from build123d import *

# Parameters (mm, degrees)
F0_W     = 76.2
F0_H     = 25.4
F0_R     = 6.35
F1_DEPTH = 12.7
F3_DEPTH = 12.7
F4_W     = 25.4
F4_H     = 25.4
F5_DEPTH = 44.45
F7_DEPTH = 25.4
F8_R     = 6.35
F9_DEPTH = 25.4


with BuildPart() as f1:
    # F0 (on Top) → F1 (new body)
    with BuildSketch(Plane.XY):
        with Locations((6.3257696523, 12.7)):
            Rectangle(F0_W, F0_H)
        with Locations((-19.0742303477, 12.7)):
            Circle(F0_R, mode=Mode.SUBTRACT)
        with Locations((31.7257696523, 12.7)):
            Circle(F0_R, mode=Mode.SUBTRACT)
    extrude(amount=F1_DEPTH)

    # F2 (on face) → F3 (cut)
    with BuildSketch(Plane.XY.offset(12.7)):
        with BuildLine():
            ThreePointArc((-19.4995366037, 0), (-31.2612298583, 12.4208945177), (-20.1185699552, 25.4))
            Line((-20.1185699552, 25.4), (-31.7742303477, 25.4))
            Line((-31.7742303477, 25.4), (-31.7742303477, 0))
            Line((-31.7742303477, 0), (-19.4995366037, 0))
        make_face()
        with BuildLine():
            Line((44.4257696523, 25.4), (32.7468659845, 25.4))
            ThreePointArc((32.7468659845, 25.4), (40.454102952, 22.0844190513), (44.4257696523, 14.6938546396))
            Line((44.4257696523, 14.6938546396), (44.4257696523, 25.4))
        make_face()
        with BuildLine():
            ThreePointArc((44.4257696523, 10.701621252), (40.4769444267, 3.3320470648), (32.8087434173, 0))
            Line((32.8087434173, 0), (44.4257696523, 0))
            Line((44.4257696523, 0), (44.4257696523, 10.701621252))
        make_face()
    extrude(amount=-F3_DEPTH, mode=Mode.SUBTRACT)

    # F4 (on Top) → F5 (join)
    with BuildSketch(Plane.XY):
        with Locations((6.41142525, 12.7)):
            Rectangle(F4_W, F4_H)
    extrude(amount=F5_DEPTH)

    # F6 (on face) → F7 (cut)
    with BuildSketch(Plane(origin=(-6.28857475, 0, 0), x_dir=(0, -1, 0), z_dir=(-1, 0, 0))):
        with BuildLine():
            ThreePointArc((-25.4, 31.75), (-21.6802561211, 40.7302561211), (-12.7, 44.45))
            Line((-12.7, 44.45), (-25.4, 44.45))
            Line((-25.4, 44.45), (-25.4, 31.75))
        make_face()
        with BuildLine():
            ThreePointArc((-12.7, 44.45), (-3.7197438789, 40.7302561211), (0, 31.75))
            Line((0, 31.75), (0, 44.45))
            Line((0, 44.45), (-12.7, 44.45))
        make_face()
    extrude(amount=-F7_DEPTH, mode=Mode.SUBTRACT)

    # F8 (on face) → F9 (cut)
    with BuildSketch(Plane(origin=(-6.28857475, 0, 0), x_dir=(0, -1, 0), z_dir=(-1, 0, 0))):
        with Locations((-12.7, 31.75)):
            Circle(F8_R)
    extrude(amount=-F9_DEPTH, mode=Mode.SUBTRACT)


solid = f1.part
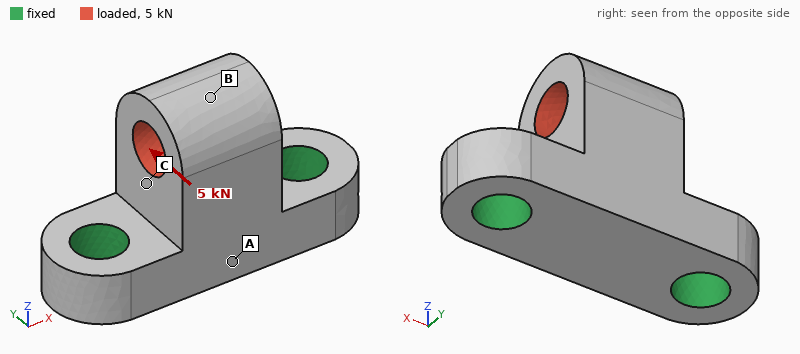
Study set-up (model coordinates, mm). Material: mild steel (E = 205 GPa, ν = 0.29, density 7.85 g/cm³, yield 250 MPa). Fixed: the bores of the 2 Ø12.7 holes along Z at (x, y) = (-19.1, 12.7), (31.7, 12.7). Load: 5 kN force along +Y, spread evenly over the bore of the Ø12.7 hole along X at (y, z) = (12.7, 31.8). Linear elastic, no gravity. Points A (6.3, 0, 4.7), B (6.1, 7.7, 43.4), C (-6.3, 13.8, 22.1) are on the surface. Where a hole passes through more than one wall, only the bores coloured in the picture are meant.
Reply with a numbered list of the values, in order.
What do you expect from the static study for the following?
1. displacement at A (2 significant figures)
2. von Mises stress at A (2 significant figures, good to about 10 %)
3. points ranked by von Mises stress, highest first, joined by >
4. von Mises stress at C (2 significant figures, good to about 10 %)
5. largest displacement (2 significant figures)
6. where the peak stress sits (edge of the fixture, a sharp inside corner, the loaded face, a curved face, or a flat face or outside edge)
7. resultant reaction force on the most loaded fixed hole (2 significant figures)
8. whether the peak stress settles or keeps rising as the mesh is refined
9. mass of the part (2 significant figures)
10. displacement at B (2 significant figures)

1. 8.8 µm
2. 18 MPa
3. C > A > B
4. 39 MPa
5. 37 µm
6. edge of the fixture
7. 2.5 kN
8. keeps rising
9. 270 g
10. 36 µm
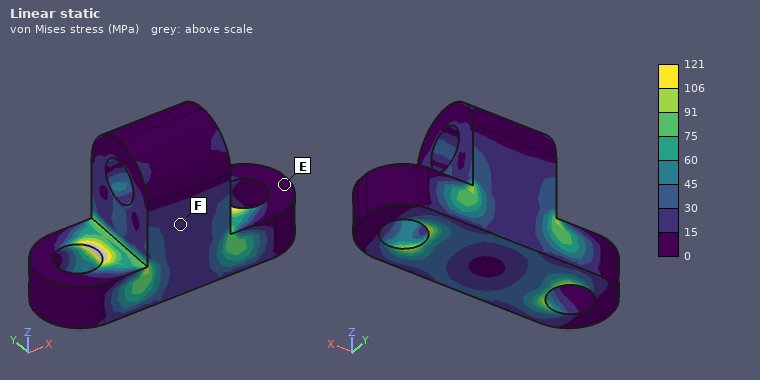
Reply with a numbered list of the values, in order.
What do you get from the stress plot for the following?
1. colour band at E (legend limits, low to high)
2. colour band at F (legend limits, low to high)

1. 0 to 15 MPa
2. 15 to 30 MPa
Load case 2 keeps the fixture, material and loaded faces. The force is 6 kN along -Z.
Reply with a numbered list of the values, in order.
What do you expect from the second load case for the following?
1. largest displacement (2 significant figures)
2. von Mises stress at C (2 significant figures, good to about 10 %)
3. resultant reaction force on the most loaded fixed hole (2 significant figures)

1. 4.6 µm
2. 8.0 MPa
3. 3.1 kN
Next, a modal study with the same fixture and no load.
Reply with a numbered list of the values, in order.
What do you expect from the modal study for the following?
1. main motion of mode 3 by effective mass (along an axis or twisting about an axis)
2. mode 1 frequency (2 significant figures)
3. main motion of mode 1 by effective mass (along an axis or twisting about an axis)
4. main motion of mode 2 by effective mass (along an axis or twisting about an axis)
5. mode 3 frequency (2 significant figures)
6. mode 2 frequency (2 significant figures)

1. along Z
2. 7100 Hz
3. along Y
4. along X
5. 17 kHz
6. 12 kHz
